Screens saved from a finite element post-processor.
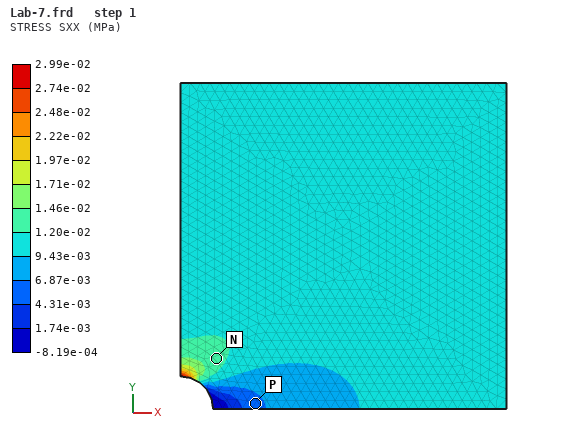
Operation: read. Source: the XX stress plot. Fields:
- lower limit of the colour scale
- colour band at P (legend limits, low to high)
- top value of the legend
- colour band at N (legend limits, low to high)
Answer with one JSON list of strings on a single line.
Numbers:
["-8.19e-04 MPa", "4.31e-03 to 6.87e-03 MPa", "2.99e-02 MPa", "1.20e-02 to 1.46e-02 MPa"]
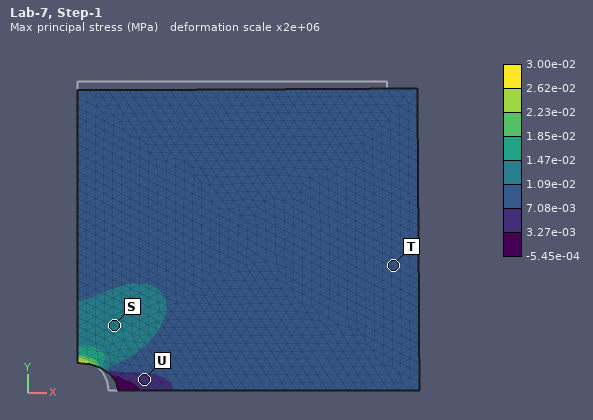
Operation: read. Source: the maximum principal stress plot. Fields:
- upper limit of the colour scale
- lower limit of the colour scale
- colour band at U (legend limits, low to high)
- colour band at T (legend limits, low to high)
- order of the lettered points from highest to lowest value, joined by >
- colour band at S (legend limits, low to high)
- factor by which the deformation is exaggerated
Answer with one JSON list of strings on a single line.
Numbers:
["3.00e-02 MPa", "-5.45e-04 MPa", "3.27e-03 to 7.08e-03 MPa", "7.08e-03 to 1.09e-02 MPa", "S > T > U", "1.09e-02 to 1.47e-02 MPa", "2e+06"]
